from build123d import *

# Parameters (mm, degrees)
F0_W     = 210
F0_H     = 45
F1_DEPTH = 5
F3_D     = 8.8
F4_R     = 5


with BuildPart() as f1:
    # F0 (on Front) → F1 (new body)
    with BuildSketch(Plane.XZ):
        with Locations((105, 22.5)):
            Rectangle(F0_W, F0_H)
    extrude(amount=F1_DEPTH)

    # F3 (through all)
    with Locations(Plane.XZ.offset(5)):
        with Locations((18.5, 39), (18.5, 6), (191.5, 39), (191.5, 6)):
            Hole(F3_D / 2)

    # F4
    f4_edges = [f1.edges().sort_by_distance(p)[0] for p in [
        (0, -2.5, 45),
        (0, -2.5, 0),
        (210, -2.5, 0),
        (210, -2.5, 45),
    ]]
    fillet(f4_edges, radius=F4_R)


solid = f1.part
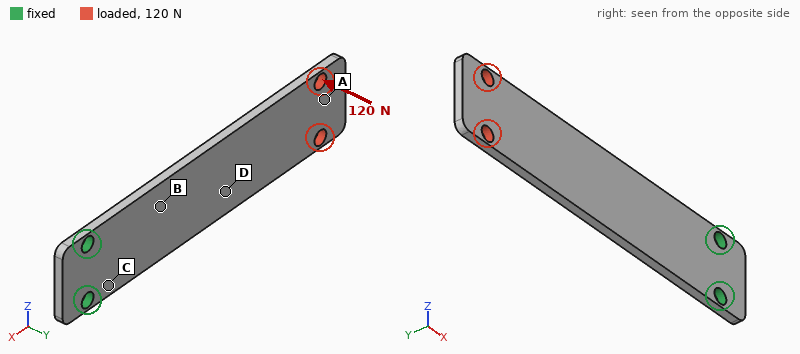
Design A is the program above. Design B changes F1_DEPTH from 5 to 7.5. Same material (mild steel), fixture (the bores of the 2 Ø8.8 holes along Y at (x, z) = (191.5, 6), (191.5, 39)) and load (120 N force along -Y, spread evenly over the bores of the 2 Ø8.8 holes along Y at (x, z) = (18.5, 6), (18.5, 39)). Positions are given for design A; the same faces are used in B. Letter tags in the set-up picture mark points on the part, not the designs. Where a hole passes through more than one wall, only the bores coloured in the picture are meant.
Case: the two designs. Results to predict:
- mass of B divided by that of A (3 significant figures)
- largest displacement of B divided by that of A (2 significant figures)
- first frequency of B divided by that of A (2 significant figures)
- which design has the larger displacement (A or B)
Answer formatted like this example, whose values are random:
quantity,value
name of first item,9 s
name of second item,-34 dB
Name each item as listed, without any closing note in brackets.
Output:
quantity,value
mass of B divided by that of A,1.50
largest displacement of B divided by that of A,0.30
first frequency of B divided by that of A,1.5
which design has the larger displacement,A
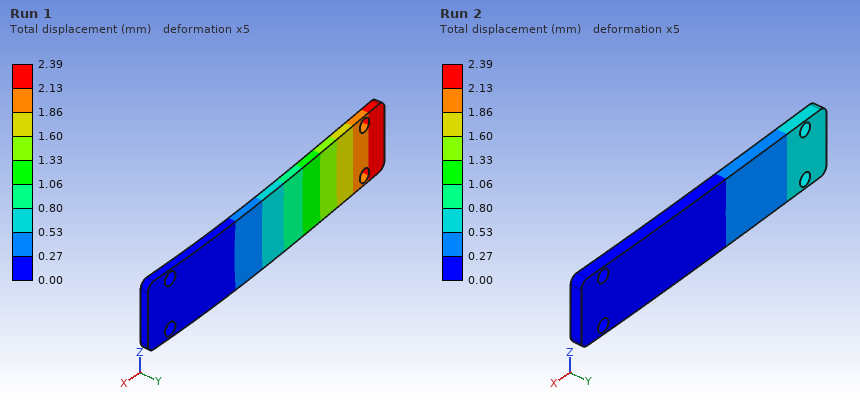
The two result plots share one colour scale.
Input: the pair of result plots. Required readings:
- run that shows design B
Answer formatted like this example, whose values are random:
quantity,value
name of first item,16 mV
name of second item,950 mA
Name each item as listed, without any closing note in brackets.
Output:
quantity,value
run that shows design B,Run 2
